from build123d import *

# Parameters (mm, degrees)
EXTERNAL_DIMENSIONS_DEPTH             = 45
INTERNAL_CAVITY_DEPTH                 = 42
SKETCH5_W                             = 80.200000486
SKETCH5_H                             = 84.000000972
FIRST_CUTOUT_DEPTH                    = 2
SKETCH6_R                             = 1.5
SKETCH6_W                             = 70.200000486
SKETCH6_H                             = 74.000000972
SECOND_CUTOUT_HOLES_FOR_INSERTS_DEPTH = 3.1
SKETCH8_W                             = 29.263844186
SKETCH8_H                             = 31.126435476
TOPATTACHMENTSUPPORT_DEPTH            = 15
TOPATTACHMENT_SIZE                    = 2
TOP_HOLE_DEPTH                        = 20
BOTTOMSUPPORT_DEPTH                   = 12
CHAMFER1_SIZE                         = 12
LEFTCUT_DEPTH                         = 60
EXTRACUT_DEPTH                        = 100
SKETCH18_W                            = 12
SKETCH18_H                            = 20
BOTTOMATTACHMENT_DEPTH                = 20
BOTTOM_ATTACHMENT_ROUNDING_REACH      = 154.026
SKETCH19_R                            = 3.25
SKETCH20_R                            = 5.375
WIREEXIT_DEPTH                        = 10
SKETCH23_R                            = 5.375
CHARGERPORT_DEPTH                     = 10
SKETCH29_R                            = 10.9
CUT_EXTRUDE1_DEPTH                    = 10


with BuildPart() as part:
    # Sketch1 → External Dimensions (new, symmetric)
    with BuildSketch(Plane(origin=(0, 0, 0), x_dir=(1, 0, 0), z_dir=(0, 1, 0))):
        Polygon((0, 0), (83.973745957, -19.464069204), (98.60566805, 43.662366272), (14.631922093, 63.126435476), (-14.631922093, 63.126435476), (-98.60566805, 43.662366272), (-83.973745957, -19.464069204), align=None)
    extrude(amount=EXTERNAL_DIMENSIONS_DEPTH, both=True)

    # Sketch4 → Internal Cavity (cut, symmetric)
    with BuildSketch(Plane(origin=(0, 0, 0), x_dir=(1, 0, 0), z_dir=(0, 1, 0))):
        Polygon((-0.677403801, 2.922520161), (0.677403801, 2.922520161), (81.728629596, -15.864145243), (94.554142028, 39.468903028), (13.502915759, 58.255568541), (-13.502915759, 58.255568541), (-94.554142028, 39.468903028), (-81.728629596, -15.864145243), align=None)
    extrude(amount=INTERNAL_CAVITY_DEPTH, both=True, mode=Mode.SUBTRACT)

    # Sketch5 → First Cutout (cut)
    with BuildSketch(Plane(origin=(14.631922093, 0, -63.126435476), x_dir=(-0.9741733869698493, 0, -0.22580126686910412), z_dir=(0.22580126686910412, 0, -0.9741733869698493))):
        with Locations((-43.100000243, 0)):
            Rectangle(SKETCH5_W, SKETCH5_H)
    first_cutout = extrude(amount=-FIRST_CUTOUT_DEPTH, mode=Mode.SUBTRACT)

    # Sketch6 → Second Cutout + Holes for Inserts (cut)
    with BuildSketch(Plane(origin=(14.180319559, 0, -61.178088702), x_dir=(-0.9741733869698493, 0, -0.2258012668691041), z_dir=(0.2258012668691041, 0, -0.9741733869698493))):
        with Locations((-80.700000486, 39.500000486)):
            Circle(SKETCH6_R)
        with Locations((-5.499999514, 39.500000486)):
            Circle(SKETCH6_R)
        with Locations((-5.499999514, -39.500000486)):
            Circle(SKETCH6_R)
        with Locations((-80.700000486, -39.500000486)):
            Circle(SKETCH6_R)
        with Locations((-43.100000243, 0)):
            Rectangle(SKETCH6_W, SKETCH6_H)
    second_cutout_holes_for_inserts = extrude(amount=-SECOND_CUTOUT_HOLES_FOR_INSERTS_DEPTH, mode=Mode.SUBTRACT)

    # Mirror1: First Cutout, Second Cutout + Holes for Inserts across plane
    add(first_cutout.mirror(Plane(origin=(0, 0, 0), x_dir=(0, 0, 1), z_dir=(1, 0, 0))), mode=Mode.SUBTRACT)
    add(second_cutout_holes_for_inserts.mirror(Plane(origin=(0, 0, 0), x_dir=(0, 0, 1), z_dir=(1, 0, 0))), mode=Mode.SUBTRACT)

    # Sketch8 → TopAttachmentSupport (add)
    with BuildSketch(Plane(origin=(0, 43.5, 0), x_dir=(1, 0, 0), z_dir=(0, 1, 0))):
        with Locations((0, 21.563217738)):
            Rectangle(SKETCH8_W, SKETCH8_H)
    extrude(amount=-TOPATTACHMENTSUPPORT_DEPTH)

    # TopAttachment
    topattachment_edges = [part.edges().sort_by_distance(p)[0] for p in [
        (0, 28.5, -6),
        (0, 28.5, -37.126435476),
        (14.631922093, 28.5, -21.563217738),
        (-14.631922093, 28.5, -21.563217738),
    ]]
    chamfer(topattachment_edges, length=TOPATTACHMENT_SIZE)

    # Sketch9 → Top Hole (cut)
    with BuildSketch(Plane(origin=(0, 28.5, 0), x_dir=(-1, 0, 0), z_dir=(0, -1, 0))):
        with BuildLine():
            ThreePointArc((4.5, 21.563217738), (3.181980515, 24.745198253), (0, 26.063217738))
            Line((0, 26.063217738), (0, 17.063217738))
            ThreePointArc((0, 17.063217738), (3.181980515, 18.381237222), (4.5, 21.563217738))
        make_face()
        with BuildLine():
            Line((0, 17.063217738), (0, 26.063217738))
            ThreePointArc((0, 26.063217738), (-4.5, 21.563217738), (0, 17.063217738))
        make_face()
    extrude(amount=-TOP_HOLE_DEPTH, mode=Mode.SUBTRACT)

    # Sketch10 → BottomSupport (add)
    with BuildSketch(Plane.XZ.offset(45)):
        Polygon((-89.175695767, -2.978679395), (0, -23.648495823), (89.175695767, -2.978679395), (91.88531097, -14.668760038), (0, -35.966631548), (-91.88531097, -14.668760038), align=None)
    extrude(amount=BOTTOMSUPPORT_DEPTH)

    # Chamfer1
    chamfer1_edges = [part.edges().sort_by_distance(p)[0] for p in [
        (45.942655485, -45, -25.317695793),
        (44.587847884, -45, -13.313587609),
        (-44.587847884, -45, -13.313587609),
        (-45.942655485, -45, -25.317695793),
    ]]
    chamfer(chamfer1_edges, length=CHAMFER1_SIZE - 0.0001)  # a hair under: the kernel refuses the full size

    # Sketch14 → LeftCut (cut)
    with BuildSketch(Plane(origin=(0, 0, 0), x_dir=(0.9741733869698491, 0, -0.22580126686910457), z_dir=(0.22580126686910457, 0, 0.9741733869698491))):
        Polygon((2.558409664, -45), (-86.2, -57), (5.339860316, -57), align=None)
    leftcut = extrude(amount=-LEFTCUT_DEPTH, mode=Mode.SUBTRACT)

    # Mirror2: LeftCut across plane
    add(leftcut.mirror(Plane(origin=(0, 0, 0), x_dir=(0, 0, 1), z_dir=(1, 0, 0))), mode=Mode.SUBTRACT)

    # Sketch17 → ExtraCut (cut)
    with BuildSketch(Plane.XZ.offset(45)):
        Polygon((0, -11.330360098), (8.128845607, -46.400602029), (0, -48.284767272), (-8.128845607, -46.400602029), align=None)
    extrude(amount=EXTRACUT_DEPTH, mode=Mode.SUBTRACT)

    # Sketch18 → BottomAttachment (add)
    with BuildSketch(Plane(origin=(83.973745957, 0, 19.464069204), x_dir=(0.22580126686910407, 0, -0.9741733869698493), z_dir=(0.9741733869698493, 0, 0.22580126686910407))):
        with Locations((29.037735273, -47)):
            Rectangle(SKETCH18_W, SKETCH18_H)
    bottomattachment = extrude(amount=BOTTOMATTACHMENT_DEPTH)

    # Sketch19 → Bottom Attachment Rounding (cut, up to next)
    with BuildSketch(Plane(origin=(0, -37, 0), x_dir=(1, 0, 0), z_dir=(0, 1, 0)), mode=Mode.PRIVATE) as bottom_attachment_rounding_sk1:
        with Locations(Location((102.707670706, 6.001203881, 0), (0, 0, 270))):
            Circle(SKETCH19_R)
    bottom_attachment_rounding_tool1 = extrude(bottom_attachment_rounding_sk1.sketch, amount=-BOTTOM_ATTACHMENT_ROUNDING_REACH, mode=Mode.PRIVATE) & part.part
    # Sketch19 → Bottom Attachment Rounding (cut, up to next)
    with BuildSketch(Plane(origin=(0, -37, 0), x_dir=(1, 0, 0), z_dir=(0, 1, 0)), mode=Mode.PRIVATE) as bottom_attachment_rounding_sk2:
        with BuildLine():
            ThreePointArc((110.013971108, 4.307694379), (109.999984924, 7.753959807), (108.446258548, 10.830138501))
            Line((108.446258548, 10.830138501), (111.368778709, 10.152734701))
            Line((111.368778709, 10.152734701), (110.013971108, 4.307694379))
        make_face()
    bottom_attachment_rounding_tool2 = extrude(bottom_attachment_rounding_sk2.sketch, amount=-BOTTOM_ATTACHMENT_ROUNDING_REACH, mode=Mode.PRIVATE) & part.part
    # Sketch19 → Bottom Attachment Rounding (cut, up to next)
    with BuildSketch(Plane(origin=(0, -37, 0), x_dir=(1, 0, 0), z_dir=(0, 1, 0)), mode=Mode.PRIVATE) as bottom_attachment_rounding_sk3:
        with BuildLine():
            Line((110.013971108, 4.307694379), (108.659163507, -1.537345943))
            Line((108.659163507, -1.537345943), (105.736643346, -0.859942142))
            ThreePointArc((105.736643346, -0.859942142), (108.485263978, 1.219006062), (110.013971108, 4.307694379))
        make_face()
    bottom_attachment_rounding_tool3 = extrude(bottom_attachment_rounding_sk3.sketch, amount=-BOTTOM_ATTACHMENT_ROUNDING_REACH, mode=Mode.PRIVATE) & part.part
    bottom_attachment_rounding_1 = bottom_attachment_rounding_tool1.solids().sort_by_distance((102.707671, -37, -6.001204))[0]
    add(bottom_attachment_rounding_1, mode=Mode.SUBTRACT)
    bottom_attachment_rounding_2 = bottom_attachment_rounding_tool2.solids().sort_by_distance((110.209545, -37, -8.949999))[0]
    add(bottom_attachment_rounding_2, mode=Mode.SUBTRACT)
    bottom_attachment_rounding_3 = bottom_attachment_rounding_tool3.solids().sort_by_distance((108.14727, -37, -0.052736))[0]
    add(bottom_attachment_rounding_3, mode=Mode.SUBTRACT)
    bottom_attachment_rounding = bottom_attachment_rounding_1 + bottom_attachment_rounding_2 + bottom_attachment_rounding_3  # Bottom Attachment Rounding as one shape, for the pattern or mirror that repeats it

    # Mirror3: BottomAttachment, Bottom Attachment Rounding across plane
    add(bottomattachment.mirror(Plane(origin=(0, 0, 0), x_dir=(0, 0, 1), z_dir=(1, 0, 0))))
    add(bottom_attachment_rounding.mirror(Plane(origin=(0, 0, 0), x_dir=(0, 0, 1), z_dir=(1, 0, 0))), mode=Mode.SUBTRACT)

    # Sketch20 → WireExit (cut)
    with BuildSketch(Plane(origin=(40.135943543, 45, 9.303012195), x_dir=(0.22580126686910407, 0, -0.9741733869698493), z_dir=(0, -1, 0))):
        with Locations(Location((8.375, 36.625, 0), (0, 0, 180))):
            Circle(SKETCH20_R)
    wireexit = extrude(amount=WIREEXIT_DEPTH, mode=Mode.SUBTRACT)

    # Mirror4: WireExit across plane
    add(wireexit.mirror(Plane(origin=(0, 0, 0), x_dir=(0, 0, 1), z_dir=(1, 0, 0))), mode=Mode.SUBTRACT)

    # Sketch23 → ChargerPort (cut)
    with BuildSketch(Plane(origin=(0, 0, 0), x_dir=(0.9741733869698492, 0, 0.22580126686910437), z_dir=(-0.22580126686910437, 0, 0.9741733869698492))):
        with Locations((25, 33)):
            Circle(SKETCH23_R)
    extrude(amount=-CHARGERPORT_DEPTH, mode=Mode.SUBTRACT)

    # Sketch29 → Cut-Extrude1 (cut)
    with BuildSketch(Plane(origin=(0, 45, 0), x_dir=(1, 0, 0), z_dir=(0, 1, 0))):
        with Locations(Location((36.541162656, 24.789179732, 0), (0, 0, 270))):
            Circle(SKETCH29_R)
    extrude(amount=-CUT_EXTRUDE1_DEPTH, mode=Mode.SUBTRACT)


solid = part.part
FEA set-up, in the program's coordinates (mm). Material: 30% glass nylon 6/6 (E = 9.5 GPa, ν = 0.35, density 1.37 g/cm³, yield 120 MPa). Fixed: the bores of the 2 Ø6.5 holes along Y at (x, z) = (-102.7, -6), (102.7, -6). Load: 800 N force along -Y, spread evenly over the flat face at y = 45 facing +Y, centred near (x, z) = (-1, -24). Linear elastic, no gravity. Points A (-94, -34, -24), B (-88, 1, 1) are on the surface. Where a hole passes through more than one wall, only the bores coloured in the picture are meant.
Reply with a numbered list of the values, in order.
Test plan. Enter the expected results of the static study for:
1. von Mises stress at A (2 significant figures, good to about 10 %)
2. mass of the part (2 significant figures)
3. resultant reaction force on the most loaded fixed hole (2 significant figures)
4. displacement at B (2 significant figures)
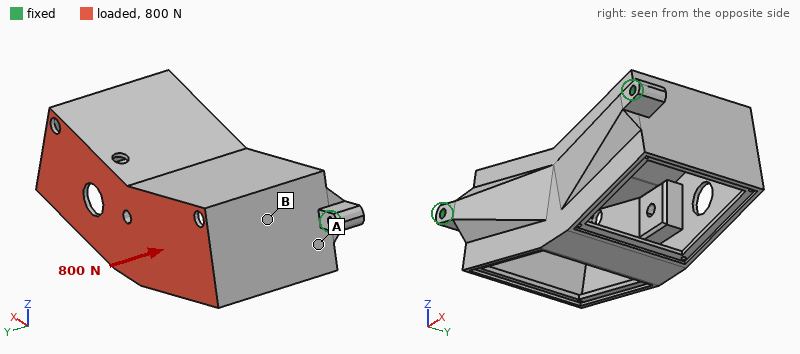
1. 4.3 MPa
2. 300 g
3. 470 N
4. 0.12 mm
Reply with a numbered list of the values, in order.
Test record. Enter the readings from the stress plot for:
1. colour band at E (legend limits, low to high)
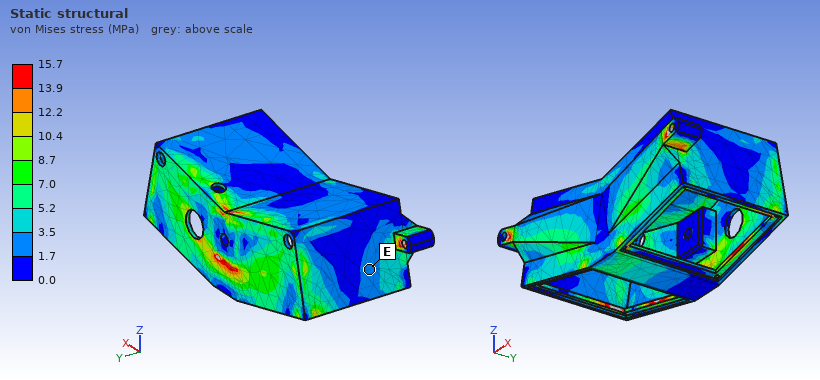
1. 1.7 to 3.5 MPa
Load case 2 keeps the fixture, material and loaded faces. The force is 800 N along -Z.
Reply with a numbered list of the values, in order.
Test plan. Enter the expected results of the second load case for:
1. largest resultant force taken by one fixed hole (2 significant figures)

1. 410 N
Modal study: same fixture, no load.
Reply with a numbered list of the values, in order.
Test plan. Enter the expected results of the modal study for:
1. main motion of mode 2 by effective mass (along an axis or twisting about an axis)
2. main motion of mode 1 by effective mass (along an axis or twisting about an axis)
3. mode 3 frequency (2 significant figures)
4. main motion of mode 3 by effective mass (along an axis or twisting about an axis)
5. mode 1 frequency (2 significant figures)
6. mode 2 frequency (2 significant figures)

1. along X
2. along Z
3. 560 Hz
4. along Y
5. 290 Hz
6. 500 Hz
